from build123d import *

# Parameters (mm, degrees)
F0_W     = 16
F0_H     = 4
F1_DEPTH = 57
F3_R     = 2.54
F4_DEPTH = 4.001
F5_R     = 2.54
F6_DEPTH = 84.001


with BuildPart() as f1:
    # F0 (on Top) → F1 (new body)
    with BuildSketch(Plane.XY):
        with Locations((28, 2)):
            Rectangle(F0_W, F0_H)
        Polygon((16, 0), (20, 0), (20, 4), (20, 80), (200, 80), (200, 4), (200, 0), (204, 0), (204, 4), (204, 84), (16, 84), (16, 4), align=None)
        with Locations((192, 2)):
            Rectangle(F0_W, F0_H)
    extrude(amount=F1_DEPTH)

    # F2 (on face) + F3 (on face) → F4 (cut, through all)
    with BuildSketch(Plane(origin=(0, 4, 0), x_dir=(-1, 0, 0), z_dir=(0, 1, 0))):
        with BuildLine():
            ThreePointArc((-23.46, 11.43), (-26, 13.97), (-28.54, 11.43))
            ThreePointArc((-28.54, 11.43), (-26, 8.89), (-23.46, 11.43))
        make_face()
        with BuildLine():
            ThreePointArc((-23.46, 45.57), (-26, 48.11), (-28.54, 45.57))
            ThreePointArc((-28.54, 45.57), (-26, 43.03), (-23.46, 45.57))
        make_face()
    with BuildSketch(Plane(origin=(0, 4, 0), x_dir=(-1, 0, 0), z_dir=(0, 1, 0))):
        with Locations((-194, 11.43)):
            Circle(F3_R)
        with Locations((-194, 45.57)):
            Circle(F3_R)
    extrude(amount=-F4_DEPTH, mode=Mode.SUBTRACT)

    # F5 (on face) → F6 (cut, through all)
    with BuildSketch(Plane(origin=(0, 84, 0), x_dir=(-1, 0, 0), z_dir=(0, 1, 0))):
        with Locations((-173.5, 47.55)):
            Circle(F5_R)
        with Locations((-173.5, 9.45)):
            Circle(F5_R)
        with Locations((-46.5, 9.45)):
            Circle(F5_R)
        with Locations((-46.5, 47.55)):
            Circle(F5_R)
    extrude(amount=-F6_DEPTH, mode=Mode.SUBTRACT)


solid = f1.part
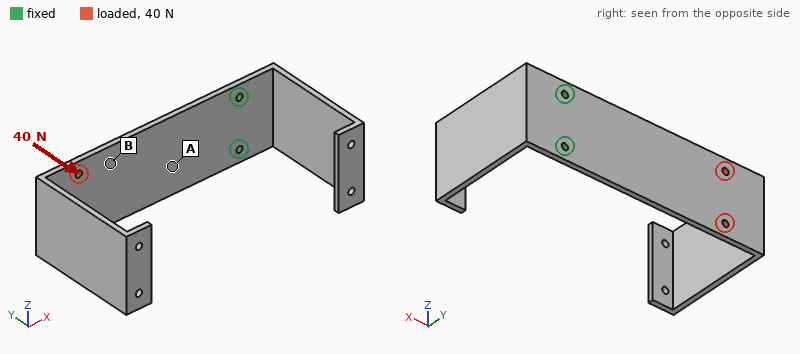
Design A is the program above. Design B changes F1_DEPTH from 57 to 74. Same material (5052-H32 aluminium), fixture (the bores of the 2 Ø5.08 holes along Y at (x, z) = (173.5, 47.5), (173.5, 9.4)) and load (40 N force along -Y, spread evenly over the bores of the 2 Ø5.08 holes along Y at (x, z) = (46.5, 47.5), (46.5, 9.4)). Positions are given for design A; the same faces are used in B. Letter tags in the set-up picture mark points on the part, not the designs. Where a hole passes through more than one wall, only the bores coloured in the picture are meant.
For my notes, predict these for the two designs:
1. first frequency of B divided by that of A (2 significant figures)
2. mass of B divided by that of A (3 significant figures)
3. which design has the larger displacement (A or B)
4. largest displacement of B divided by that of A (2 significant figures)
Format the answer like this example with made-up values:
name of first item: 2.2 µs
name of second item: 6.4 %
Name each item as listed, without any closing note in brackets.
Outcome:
first frequency of B divided by that of A: 0.99
mass of B divided by that of A: 1.30
which design has the larger displacement: A
largest displacement of B divided by that of A: 0.79
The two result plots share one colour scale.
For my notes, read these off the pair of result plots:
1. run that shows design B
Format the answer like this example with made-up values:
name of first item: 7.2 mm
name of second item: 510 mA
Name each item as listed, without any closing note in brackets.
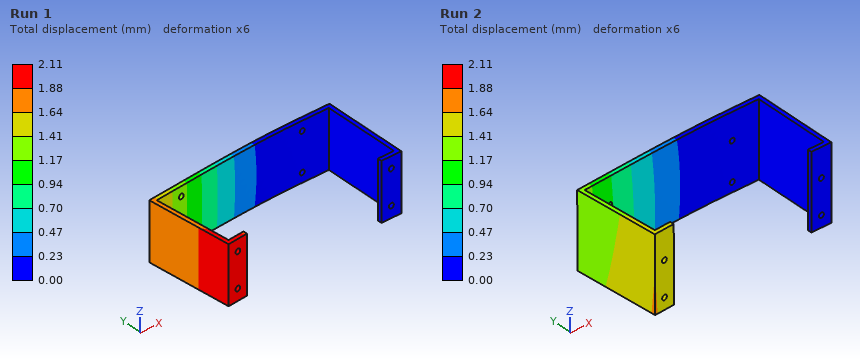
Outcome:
run that shows design B: Run 2
